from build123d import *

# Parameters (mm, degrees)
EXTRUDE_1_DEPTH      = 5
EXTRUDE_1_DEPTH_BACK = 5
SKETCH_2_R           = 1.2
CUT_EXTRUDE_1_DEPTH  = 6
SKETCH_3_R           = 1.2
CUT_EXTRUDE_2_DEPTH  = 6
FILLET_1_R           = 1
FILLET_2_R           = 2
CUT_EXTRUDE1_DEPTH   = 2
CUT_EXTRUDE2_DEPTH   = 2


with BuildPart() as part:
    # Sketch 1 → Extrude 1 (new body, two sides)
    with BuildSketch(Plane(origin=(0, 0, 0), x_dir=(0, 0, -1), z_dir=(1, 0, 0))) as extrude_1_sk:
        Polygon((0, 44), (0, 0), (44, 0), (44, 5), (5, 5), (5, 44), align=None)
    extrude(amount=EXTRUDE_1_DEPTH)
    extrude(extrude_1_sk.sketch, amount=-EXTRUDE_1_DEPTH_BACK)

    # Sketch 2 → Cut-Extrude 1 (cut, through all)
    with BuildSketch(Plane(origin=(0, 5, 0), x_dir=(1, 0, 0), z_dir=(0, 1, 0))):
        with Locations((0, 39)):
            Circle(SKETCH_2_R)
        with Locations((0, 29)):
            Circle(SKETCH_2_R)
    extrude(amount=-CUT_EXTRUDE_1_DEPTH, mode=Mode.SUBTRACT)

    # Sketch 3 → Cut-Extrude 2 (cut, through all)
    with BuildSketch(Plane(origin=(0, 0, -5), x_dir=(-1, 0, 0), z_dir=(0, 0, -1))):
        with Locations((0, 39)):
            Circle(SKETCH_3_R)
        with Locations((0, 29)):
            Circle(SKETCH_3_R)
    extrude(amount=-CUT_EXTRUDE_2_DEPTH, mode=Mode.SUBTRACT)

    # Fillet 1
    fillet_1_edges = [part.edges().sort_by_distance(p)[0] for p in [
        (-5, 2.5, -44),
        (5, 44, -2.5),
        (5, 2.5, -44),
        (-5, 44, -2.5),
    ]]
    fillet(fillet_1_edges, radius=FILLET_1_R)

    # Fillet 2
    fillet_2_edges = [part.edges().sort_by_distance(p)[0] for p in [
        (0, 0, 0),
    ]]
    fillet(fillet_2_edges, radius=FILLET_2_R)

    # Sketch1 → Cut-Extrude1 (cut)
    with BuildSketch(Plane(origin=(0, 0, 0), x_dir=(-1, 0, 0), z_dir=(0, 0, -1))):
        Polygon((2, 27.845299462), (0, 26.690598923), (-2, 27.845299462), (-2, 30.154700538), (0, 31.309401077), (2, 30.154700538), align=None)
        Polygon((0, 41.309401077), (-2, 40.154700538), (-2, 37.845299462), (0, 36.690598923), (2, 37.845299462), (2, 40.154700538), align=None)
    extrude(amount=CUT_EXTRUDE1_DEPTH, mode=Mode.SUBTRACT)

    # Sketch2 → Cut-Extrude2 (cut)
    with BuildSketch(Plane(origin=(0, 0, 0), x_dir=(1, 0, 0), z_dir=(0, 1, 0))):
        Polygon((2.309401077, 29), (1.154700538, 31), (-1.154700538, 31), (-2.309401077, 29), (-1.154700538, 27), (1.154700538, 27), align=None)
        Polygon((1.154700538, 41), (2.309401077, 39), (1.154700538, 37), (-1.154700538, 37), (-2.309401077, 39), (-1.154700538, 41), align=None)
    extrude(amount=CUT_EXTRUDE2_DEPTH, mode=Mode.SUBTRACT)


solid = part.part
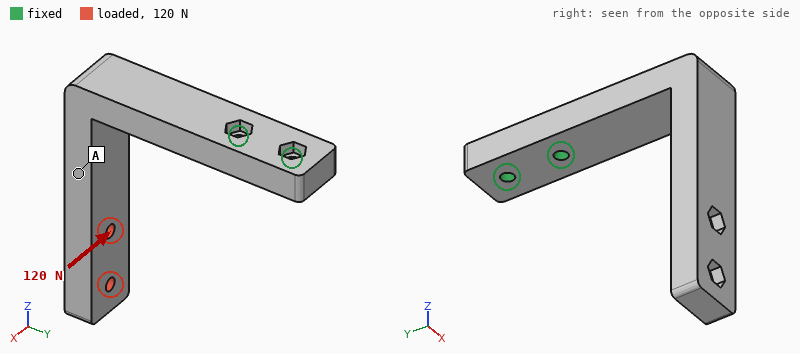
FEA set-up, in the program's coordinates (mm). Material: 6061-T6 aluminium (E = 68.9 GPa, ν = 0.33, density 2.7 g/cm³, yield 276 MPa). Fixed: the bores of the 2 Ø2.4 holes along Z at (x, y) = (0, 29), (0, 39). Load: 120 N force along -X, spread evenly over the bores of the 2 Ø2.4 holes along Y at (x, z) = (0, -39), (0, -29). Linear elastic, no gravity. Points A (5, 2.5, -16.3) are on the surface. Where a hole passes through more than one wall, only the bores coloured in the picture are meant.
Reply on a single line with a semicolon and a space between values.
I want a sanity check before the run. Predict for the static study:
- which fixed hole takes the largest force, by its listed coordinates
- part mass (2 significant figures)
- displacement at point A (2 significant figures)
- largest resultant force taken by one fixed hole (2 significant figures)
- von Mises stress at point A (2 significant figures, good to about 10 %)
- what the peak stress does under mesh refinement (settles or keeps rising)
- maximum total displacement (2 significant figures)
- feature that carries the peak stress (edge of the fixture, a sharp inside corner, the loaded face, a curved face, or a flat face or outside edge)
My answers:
(0, 29); 11 g; 0.25 mm; 360 N; 25 MPa; keeps rising; 0.69 mm; edge of the fixture
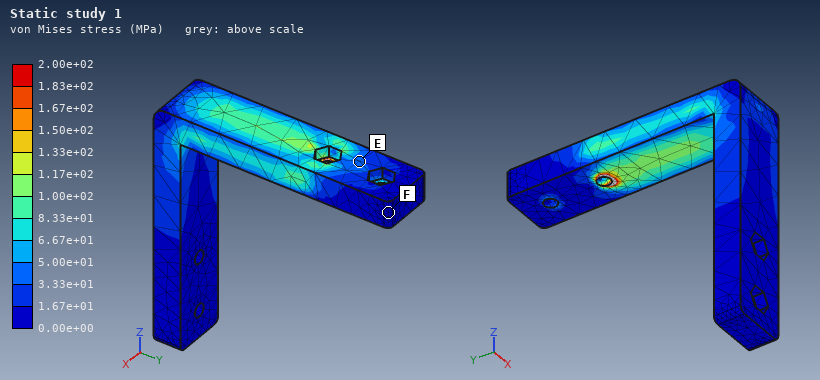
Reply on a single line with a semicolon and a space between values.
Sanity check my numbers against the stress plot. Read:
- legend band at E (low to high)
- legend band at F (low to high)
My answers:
3.33e+01 to 5.00e+01 MPa; 0.00e+00 to 1.67e+01 MPa
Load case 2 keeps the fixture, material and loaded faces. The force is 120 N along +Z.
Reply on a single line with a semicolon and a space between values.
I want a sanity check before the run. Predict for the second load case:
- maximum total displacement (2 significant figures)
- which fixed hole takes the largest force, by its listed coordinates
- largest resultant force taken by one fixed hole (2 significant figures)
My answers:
0.30 mm; (0, 29); 350 N
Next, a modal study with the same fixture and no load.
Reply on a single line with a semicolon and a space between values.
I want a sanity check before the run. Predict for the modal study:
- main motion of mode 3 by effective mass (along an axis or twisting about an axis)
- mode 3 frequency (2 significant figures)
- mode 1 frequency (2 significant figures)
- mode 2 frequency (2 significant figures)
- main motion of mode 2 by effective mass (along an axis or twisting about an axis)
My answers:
along Z; 3200 Hz; 1100 Hz; 1400 Hz; along X
